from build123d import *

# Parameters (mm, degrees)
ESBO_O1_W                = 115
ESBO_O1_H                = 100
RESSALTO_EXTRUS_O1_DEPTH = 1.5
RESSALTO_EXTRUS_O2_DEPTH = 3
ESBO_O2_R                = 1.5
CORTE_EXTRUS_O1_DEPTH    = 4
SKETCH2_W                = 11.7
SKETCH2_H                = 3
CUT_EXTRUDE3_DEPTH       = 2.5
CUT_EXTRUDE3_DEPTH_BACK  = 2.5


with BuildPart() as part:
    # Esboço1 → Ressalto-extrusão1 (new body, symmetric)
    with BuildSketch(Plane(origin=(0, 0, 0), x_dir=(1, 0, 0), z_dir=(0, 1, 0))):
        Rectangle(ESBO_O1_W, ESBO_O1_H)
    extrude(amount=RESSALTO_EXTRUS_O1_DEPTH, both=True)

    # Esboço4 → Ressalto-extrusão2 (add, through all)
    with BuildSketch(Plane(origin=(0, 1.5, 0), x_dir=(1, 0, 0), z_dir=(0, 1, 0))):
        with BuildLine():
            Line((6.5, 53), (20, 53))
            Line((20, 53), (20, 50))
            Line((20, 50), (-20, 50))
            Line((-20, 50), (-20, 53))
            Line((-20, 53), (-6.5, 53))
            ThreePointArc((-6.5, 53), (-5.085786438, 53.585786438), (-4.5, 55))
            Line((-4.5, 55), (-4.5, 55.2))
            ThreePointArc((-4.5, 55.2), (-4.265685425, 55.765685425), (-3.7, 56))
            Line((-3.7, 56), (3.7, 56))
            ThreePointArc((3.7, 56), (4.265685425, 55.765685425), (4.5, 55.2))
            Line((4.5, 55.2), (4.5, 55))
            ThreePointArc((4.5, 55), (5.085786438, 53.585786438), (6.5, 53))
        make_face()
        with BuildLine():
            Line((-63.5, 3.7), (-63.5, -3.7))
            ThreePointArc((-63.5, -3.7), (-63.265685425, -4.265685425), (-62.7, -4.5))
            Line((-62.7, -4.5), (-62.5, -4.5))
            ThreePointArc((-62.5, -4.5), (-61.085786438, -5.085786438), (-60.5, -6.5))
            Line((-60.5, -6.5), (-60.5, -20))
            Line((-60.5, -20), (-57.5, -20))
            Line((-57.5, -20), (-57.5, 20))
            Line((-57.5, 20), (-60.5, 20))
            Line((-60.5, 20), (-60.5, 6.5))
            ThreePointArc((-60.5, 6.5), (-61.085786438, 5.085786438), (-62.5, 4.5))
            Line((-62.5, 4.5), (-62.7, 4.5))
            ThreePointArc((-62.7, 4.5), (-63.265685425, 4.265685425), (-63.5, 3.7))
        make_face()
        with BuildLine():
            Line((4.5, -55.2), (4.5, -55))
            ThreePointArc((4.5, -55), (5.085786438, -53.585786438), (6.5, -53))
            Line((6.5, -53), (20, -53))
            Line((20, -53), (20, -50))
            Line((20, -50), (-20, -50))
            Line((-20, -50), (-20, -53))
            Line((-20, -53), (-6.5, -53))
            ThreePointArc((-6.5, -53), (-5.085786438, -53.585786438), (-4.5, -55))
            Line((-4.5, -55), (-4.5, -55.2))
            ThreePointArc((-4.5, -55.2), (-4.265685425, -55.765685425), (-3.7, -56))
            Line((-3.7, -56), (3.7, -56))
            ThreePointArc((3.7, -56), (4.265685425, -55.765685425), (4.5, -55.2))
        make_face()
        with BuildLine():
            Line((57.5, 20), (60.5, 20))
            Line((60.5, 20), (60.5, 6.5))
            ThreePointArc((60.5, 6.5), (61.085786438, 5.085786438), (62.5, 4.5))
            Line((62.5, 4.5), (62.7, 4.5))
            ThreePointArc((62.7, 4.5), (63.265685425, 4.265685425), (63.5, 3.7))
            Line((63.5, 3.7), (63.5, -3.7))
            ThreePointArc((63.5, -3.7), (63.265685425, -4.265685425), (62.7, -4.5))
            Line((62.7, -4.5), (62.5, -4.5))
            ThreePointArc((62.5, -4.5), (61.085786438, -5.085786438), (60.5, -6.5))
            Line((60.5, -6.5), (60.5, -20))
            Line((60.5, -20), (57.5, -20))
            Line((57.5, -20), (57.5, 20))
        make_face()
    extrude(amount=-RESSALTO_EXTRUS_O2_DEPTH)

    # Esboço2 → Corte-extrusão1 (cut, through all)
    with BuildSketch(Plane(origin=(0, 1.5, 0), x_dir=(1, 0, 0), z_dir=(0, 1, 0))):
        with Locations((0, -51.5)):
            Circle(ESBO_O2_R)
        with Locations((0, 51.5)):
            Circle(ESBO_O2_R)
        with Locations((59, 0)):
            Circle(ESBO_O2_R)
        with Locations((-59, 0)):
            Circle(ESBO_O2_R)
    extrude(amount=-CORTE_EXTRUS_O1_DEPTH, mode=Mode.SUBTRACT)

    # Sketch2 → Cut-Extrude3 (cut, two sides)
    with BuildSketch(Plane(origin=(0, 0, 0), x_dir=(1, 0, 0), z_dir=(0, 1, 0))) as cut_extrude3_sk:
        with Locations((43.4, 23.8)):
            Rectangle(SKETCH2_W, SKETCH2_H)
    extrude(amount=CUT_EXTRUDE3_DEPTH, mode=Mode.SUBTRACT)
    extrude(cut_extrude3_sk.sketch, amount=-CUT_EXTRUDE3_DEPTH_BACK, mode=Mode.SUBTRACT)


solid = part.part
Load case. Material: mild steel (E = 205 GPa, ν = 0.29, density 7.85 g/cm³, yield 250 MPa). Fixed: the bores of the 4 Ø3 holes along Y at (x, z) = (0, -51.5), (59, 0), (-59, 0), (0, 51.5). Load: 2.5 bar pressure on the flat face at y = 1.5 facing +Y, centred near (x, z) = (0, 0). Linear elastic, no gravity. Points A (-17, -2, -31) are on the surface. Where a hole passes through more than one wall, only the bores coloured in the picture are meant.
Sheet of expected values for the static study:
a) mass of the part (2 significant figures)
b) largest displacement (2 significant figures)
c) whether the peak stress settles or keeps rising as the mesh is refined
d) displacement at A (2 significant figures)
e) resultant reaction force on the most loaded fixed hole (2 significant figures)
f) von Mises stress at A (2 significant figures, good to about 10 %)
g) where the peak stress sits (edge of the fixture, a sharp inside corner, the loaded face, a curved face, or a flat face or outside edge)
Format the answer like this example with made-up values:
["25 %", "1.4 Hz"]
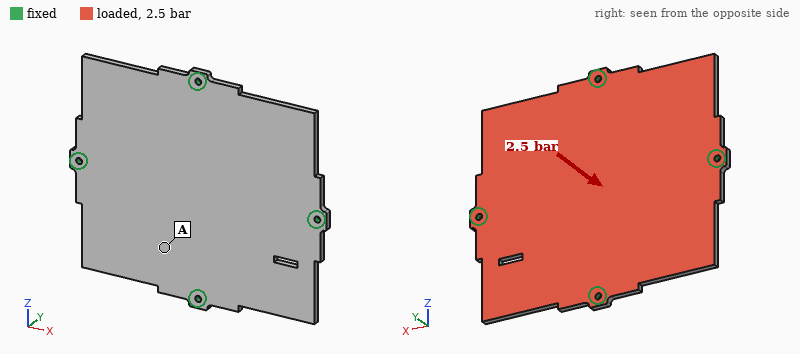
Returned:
["280 g", "0.14 mm", "keeps rising", "0.084 mm", "770 N", "55 MPa", "edge of the fixture"]
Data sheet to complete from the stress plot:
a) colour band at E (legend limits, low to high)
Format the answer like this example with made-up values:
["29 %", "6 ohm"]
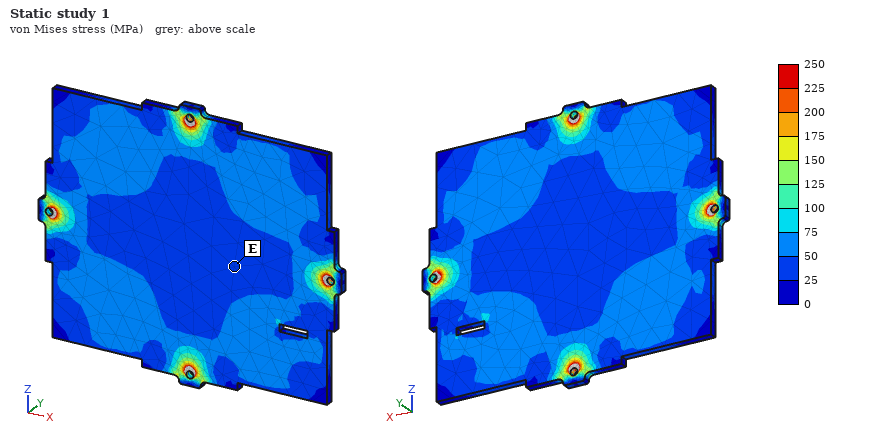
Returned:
["25 to 50 MPa"]
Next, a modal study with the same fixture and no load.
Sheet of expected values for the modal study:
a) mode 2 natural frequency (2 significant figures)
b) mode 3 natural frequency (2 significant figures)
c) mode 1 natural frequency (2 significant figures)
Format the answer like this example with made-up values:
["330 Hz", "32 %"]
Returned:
["1600 Hz", "1700 Hz", "1500 Hz"]
